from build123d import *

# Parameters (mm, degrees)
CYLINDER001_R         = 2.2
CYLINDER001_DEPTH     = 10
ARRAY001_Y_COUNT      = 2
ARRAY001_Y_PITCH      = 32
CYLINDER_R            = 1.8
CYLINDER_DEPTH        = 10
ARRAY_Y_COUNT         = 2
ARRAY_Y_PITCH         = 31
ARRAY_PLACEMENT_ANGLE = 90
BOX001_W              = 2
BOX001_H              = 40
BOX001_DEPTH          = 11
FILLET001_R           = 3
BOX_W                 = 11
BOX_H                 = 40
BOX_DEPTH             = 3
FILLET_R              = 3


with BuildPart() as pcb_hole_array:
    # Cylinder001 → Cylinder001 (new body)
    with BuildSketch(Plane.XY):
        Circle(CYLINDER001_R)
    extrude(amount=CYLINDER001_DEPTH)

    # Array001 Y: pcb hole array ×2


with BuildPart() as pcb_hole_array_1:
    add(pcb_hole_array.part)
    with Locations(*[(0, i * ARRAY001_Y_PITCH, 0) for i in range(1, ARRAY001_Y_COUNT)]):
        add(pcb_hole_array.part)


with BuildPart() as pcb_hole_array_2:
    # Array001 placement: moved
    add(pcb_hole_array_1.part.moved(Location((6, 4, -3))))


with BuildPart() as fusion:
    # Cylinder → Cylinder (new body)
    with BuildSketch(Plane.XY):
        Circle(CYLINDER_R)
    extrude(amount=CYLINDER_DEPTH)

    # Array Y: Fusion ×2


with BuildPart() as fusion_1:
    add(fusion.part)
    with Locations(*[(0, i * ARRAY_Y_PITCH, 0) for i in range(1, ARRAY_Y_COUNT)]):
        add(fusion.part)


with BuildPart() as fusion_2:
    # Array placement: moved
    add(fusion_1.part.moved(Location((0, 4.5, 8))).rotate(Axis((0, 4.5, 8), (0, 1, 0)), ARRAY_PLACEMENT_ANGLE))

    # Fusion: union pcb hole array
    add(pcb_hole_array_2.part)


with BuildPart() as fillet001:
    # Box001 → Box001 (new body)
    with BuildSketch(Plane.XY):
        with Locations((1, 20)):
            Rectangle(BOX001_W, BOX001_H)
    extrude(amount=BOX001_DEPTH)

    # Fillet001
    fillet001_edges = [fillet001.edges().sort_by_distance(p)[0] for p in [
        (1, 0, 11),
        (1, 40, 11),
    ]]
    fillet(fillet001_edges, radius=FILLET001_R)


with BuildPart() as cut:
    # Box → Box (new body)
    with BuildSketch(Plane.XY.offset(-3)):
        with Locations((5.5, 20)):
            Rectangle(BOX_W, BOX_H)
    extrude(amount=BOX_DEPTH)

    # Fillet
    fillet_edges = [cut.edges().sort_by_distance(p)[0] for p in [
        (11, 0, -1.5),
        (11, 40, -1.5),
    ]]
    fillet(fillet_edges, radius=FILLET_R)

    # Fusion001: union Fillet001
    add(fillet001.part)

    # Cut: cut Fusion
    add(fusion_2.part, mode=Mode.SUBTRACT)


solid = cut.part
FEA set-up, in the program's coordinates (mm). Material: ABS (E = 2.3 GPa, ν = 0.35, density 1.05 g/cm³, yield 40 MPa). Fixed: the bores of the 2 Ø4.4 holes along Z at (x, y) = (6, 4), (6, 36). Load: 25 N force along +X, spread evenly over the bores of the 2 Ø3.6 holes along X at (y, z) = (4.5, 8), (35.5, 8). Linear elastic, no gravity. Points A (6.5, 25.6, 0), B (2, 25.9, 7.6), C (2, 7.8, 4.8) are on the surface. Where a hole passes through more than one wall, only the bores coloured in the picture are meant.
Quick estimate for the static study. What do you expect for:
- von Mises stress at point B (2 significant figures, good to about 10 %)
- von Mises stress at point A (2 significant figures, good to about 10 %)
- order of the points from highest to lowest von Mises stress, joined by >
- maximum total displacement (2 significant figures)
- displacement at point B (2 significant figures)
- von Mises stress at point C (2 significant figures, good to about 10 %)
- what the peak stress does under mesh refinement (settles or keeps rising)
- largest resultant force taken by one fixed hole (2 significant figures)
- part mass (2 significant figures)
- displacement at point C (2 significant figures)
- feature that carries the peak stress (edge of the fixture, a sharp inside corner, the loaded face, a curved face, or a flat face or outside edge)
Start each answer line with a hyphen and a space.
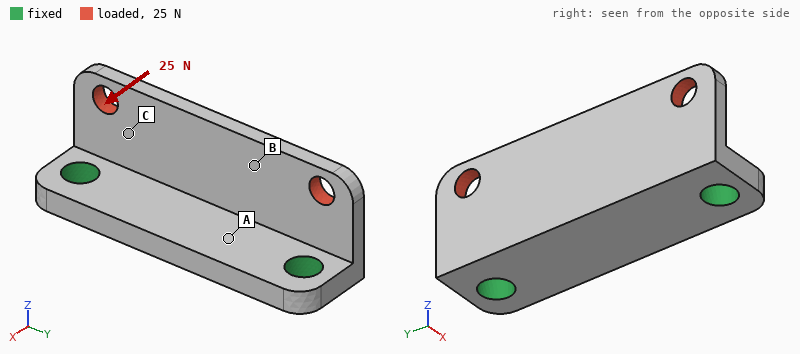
- 2.7 MPa
- 1.3 MPa
- C > B > A
- 0.27 mm
- 0.11 mm
- 4.4 MPa
- keeps rising
- 13 N
- 2.2 g
- 0.085 mm
- edge of the fixture
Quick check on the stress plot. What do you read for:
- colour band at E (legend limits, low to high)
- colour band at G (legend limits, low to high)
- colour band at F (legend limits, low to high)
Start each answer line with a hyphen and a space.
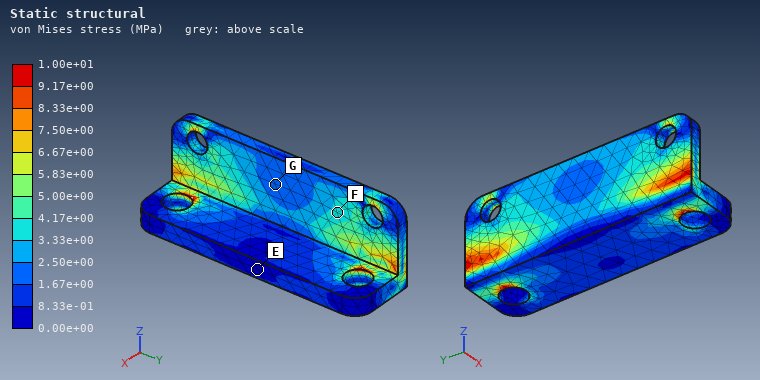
- 0.00e+00 to 8.33e-01 MPa
- 1.67e+00 to 2.50e+00 MPa
- 3.33e+00 to 4.17e+00 MPa
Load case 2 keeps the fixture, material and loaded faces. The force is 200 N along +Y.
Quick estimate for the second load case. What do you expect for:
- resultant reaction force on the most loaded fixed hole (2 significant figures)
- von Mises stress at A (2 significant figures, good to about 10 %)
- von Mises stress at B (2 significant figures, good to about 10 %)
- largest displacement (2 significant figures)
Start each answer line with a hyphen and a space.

- 120 N
- 2.0 MPa
- 4.7 MPa
- 0.12 mm
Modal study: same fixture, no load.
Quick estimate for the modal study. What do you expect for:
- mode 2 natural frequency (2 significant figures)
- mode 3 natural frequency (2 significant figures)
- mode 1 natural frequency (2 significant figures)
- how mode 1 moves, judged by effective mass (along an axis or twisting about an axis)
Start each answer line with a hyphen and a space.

- 3900 Hz
- 5600 Hz
- 2700 Hz
- along X
